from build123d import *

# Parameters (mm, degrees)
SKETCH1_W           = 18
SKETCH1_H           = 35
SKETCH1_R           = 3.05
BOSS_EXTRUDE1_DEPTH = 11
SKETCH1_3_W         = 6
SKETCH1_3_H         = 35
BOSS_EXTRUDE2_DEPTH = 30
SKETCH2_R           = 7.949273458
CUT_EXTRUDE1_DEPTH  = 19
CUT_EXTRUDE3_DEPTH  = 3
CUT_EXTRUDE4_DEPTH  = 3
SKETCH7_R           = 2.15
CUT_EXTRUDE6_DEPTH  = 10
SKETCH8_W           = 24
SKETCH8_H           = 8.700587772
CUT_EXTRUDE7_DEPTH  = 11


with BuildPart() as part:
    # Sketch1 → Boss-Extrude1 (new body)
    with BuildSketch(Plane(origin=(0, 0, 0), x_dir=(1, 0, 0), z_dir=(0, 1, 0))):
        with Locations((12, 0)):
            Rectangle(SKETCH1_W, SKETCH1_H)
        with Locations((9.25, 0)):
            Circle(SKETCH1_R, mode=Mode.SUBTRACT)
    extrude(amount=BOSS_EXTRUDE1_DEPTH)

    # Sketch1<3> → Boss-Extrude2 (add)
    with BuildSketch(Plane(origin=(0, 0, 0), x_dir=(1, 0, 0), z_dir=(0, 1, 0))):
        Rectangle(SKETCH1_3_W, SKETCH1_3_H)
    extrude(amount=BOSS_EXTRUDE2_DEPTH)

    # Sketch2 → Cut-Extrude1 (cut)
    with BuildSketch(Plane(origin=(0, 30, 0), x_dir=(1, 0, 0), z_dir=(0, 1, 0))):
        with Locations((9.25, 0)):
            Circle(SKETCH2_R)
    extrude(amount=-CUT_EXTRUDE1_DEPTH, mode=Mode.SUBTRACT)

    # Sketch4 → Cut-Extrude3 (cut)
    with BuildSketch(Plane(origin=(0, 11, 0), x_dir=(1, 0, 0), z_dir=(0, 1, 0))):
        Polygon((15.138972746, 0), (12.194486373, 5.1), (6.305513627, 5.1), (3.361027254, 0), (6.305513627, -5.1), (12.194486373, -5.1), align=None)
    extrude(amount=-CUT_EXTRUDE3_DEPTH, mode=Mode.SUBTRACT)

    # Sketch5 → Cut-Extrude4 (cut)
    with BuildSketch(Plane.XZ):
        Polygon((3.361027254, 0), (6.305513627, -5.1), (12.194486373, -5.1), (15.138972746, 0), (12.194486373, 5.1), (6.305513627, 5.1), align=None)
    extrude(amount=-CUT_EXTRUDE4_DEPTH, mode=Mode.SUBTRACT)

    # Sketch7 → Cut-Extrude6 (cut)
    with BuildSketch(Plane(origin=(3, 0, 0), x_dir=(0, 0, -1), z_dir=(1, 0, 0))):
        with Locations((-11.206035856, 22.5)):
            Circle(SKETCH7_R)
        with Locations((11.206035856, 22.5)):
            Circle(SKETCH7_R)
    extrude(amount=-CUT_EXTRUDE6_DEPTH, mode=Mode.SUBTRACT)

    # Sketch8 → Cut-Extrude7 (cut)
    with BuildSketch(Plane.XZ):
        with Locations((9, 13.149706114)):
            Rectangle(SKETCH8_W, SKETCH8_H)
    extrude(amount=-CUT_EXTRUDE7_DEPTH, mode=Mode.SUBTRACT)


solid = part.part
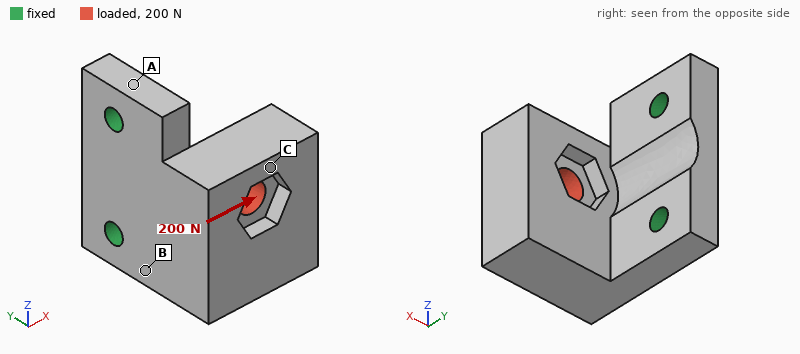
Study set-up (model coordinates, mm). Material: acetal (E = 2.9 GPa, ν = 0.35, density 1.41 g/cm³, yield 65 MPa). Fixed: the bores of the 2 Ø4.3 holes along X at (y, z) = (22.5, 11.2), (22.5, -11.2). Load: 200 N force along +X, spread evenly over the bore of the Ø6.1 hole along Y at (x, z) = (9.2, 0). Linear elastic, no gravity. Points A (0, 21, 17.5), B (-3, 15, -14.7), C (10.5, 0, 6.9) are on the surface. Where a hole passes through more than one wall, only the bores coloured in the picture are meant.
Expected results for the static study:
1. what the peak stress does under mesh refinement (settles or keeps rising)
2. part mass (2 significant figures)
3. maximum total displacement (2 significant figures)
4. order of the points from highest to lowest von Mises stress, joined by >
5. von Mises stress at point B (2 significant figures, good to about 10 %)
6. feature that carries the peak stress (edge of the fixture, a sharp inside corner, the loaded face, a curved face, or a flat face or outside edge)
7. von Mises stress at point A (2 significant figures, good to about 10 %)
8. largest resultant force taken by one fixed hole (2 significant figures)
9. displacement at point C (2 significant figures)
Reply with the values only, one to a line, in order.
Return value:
keeps rising
14 g
0.57 mm
B > A > C
12 MPa
edge of the fixture
5.2 MPa
100 N
0.43 mm
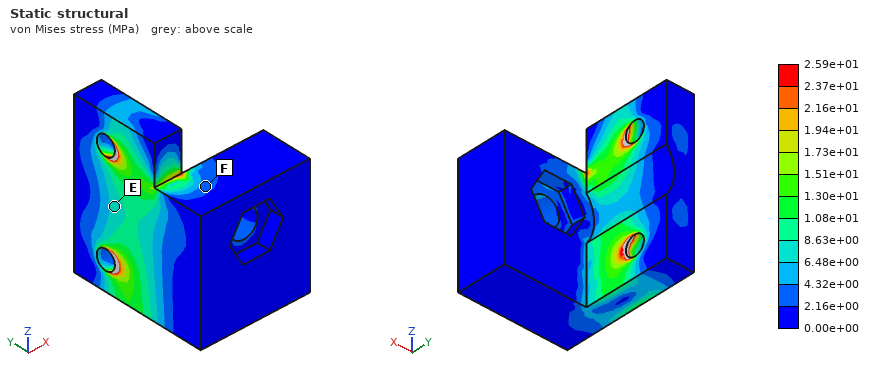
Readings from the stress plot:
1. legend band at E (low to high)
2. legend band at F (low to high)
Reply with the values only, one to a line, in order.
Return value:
6.48e+00 to 8.63e+00 MPa
2.16e+00 to 4.32e+00 MPa
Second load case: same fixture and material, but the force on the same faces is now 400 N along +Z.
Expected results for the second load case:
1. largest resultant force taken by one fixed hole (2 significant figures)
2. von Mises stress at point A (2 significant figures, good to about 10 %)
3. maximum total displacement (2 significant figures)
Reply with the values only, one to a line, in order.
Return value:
360 N
3.9 MPa
0.33 mm
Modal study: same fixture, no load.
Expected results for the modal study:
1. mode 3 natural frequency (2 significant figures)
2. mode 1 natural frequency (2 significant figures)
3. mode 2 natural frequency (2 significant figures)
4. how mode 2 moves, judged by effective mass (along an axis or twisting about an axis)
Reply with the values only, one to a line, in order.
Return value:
3700 Hz
1000 Hz
2100 Hz
along Z
